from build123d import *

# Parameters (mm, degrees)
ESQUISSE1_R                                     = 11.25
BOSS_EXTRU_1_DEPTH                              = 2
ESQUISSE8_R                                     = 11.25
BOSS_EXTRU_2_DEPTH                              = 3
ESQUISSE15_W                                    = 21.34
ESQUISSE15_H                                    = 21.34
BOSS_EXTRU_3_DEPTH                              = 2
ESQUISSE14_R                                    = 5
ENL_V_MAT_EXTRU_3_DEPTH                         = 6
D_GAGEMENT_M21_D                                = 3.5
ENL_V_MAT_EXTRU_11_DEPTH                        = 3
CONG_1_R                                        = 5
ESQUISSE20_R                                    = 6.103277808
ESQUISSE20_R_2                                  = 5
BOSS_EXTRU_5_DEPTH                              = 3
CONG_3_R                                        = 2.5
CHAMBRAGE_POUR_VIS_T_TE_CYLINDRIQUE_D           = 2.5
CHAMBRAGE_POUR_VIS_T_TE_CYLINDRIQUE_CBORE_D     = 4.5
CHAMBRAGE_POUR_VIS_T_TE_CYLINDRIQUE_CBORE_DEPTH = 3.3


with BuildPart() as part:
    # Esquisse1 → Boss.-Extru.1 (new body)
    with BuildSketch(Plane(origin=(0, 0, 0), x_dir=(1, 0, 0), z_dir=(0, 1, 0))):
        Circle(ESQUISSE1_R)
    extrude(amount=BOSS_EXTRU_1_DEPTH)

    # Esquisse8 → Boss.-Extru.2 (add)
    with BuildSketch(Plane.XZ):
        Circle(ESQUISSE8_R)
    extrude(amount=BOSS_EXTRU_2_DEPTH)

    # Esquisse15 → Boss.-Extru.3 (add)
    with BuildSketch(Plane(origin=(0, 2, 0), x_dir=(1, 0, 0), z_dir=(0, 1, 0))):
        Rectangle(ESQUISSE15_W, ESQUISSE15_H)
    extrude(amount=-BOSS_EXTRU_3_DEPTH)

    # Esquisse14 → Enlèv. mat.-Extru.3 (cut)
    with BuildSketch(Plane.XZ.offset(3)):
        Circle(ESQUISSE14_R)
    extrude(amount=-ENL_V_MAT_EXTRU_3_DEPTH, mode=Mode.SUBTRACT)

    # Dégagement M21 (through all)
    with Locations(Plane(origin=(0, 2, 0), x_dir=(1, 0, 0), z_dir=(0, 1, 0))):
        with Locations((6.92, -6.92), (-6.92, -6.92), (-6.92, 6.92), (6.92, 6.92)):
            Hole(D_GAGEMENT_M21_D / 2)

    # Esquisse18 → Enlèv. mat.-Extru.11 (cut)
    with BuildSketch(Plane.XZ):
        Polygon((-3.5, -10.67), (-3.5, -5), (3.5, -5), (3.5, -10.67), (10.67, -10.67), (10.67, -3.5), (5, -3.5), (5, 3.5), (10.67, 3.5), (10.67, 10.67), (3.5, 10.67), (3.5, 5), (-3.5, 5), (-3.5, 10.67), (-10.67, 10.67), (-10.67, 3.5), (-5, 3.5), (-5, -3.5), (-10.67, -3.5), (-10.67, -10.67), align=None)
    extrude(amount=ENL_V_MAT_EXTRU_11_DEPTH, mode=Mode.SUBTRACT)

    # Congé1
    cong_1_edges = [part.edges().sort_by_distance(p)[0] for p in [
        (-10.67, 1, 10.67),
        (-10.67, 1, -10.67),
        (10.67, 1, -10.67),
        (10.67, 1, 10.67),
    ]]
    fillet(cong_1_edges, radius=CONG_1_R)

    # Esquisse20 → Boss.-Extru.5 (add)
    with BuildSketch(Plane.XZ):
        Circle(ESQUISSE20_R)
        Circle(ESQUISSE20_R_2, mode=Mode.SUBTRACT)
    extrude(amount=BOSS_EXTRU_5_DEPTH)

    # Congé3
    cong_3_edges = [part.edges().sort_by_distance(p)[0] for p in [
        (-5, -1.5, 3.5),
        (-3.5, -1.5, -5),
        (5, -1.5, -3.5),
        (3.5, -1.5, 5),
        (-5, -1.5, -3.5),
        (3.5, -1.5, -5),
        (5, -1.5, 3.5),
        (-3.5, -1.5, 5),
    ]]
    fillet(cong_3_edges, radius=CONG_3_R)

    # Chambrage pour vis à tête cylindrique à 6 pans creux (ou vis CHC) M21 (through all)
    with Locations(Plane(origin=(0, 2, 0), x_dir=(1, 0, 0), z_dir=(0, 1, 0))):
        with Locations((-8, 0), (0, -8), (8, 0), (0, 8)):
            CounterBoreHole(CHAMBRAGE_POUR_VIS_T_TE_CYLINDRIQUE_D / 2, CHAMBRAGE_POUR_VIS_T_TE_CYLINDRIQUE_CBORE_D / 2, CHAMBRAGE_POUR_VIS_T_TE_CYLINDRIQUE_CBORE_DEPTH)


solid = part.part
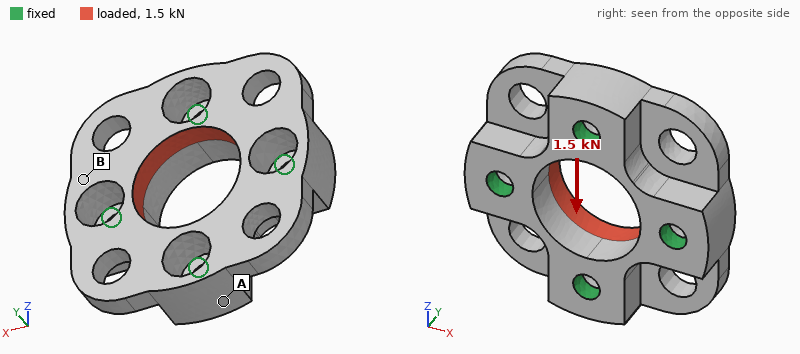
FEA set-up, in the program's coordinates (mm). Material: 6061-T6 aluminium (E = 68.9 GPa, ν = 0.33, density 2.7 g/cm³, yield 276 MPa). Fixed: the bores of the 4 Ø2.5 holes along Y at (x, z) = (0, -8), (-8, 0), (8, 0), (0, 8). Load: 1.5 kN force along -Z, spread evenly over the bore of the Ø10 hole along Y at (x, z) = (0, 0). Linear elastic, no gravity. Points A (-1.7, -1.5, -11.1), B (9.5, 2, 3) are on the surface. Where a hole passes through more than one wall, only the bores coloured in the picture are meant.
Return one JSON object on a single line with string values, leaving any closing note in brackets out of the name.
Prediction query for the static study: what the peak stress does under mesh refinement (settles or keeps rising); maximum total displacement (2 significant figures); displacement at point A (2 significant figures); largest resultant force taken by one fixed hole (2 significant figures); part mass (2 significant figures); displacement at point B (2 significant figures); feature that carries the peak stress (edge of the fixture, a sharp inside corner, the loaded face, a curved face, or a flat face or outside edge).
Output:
{"what the peak stress does under mesh refinement": "keeps rising", "maximum total displacement": "11 µm", "displacement at point A": "3.3 µm", "largest resultant force taken by one fixed hole": "460 N", "part mass": "2.6 g", "displacement at point B": "5.3 µm", "feature that carries the peak stress": "edge of the fixture"}
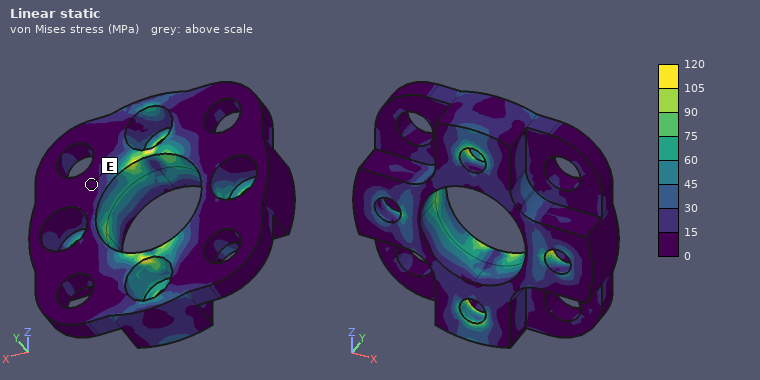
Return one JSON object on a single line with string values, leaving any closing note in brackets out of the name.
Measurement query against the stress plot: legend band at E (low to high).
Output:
{"legend band at E": "0 to 15 MPa"}
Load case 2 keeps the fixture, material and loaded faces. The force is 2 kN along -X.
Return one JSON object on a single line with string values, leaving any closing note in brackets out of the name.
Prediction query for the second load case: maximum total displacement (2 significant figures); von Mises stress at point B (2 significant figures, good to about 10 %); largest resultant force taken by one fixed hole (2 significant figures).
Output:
{"maximum total displacement": "15 µm", "von Mises stress at point B": "16 MPa", "largest resultant force taken by one fixed hole": "610 N"}
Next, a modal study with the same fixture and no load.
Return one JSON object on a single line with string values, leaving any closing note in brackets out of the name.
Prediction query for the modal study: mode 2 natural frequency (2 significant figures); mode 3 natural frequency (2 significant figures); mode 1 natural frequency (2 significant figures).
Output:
{"mode 2 natural frequency": "42 kHz", "mode 3 natural frequency": "42 kHz", "mode 1 natural frequency": "37 kHz"}
